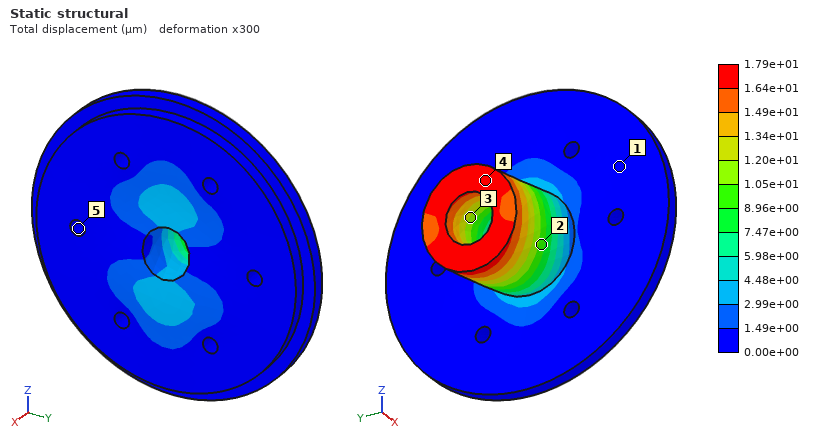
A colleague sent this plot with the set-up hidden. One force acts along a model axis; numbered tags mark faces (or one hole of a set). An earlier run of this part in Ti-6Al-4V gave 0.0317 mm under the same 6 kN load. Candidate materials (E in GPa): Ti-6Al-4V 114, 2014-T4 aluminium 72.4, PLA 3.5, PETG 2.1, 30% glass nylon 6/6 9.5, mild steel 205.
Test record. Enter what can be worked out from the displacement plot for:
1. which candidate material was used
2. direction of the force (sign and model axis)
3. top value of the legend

mild steel
-Z
1.79e+01 µm
